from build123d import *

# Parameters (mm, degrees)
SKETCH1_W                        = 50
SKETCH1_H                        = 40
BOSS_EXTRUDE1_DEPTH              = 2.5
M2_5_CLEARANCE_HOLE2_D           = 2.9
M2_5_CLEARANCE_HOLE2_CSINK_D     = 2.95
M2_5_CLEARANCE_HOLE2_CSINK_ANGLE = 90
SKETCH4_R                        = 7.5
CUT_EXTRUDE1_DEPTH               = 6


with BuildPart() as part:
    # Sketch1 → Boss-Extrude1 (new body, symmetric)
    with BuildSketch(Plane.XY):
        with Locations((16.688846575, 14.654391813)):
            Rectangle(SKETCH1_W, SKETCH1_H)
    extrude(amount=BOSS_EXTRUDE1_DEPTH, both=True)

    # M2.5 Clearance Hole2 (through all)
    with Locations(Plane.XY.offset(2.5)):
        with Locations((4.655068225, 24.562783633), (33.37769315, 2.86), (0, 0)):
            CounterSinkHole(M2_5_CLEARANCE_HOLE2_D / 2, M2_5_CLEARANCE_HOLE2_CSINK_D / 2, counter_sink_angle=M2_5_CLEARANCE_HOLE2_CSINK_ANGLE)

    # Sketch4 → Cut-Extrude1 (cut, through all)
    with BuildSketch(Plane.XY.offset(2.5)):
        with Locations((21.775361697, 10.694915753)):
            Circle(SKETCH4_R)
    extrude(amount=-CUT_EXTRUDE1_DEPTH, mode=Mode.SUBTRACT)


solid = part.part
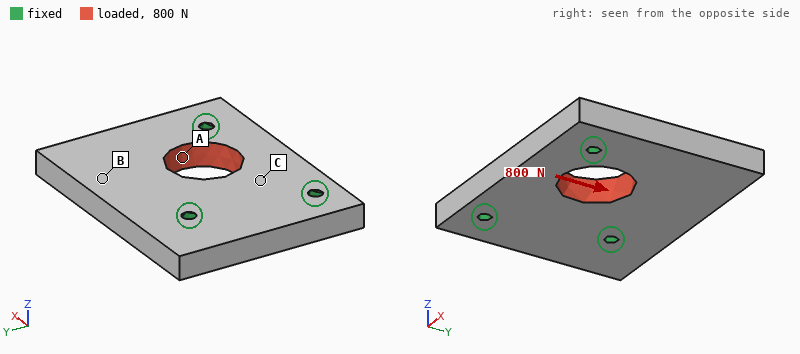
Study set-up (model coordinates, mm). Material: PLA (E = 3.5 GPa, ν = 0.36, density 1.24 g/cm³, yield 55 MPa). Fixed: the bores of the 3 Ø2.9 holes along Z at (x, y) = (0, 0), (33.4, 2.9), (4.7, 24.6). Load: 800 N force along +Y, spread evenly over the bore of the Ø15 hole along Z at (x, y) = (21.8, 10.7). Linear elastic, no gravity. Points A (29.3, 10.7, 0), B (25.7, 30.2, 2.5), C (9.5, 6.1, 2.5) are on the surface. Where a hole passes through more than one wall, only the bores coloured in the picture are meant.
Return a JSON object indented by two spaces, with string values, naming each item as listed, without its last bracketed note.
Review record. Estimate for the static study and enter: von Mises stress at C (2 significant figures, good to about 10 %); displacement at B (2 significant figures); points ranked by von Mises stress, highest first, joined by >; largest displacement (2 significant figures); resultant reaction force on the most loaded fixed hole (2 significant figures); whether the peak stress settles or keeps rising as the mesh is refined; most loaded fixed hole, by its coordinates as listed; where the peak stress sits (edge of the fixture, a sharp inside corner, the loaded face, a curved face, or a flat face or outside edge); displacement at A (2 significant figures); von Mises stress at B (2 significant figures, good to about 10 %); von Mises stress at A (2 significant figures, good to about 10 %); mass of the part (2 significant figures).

{
  "von Mises stress at C": "3.9 MPa",
  "displacement at B": "25 µm",
  "points ranked by von Mises stress, highest first, joined by >": "A > C > B",
  "largest displacement": "39 µm",
  "resultant reaction force on the most loaded fixed hole": "420 N",
  "whether the peak stress settles or keeps rising as the mesh is refined": "keeps rising",
  "most loaded fixed hole, by its coordinates as listed": "(33.4, 2.9)",
  "where the peak stress sits": "edge of the fixture",
  "displacement at A": "21 µm",
  "von Mises stress at B": "1.8 MPa",
  "von Mises stress at A": "7.8 MPa",
  "mass of the part": "11 g"
}
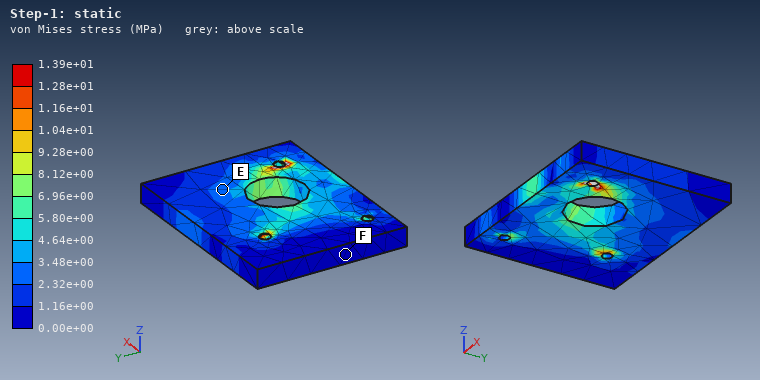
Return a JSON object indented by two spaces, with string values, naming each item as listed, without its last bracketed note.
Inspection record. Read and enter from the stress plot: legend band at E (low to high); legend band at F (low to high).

{
  "legend band at E": "2.32e+00 to 3.48e+00 MPa",
  "legend band at F": "0.00e+00 to 1.16e+00 MPa"
}
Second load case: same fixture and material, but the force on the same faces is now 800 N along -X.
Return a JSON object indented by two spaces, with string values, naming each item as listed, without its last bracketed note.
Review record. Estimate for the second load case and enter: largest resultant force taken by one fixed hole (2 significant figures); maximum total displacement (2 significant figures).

{
  "largest resultant force taken by one fixed hole": "310 N",
  "maximum total displacement": "30 µm"
}
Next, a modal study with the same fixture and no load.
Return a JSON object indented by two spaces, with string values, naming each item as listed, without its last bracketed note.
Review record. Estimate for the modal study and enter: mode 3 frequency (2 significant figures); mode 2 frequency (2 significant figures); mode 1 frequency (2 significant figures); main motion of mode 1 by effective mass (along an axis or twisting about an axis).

{
  "mode 3 frequency": "6500 Hz",
  "mode 2 frequency": "5600 Hz",
  "mode 1 frequency": "1900 Hz",
  "main motion of mode 1 by effective mass": "along Z"
}
